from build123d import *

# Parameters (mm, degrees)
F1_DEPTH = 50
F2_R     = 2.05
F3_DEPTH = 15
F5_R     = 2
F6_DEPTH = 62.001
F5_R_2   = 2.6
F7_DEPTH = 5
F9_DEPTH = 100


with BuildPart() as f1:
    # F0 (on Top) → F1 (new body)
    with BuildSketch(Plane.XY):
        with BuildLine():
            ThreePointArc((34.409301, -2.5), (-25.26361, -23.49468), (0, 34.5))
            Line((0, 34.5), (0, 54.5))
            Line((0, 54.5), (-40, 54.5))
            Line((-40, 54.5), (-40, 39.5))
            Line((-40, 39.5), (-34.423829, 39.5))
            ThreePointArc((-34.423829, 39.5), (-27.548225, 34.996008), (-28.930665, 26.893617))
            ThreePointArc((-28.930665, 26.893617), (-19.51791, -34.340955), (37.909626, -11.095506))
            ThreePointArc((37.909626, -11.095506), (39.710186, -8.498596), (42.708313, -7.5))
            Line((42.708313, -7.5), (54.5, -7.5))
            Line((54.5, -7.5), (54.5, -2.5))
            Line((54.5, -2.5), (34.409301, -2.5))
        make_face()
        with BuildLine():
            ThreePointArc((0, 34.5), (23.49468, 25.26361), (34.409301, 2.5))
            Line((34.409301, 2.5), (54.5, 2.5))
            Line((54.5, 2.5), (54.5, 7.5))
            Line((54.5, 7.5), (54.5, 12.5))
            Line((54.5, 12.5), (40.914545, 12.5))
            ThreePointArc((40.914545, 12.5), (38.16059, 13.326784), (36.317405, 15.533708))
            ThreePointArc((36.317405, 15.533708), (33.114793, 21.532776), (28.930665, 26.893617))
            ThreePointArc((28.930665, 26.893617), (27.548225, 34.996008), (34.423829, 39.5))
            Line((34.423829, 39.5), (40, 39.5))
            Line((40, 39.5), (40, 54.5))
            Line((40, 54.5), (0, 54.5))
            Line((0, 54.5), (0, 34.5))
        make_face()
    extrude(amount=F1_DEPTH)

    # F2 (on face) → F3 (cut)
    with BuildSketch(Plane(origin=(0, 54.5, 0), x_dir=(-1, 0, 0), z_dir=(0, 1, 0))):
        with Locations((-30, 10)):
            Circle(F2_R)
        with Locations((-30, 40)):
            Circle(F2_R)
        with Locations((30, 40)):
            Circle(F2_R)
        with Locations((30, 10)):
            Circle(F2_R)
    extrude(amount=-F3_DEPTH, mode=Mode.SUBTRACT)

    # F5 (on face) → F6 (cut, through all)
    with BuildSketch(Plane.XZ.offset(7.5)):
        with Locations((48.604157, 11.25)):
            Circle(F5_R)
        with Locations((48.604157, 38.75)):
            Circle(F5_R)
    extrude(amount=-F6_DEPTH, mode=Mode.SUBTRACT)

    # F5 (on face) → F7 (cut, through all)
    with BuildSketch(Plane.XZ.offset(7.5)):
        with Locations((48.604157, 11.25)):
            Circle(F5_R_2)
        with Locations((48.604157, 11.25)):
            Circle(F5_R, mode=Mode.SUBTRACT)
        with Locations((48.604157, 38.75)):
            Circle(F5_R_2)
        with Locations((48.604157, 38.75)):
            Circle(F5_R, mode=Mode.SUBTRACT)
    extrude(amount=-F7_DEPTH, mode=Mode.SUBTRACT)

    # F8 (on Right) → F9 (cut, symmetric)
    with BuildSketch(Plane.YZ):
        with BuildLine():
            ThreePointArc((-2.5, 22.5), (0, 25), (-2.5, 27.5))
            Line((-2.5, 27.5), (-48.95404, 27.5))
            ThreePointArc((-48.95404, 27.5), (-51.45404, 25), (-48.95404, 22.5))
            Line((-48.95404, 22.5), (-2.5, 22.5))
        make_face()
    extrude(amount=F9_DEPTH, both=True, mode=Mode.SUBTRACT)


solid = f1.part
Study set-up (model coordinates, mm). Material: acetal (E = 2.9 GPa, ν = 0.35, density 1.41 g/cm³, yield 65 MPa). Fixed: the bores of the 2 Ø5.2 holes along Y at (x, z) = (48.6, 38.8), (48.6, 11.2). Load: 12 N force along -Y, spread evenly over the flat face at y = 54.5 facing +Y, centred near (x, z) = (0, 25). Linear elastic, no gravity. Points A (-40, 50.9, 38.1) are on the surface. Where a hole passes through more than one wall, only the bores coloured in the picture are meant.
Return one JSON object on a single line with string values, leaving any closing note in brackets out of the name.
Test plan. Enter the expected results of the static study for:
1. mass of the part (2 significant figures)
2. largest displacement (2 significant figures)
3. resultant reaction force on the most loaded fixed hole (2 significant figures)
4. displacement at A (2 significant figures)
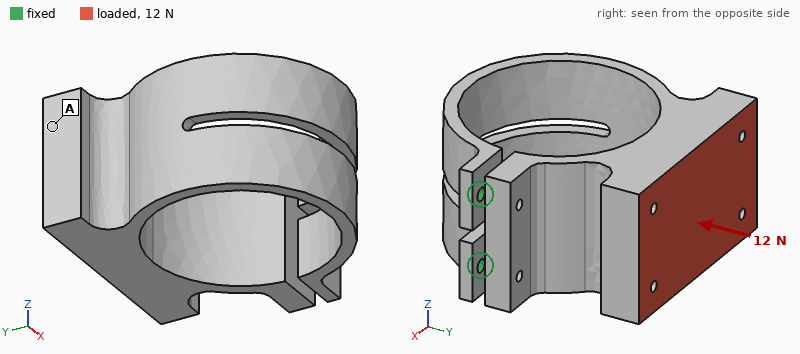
{"mass of the part": "190 g", "largest displacement": "1.4 mm", "resultant reaction force on the most loaded fixed hole": "6.0 N", "displacement at A": "0.79 mm"}
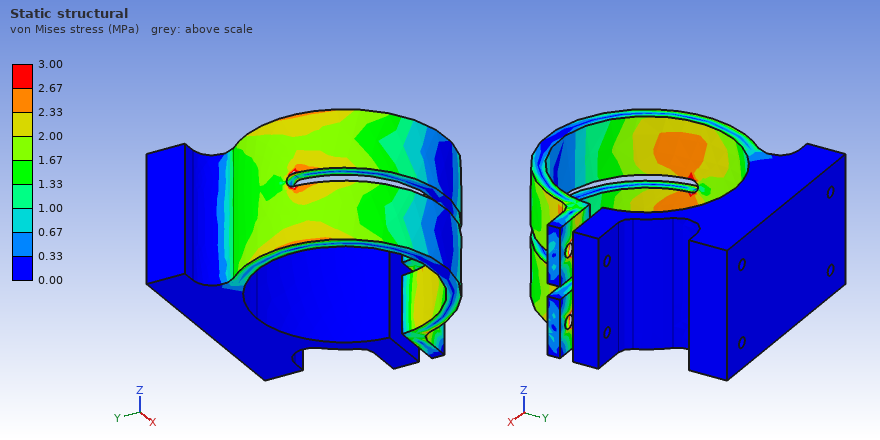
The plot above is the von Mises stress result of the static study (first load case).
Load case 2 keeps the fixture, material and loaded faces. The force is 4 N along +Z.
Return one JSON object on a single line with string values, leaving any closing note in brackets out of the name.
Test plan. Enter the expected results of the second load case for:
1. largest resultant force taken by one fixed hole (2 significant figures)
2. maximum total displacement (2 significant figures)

{"largest resultant force taken by one fixed hole": "2.3 N", "maximum total displacement": "1.5 mm"}
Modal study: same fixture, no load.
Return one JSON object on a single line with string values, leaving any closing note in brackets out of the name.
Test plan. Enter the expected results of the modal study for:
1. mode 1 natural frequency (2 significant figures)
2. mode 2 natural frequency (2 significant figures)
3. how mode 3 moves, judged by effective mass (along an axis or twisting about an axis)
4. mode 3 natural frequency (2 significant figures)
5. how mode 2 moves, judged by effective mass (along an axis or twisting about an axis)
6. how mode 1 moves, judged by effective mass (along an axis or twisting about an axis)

{"mode 1 natural frequency": "20 Hz", "mode 2 natural frequency": "26 Hz", "how mode 3 moves, judged by effective mass": "along Y", "mode 3 natural frequency": "42 Hz", "how mode 2 moves, judged by effective mass": "along Z", "how mode 1 moves, judged by effective mass": "along X"}
